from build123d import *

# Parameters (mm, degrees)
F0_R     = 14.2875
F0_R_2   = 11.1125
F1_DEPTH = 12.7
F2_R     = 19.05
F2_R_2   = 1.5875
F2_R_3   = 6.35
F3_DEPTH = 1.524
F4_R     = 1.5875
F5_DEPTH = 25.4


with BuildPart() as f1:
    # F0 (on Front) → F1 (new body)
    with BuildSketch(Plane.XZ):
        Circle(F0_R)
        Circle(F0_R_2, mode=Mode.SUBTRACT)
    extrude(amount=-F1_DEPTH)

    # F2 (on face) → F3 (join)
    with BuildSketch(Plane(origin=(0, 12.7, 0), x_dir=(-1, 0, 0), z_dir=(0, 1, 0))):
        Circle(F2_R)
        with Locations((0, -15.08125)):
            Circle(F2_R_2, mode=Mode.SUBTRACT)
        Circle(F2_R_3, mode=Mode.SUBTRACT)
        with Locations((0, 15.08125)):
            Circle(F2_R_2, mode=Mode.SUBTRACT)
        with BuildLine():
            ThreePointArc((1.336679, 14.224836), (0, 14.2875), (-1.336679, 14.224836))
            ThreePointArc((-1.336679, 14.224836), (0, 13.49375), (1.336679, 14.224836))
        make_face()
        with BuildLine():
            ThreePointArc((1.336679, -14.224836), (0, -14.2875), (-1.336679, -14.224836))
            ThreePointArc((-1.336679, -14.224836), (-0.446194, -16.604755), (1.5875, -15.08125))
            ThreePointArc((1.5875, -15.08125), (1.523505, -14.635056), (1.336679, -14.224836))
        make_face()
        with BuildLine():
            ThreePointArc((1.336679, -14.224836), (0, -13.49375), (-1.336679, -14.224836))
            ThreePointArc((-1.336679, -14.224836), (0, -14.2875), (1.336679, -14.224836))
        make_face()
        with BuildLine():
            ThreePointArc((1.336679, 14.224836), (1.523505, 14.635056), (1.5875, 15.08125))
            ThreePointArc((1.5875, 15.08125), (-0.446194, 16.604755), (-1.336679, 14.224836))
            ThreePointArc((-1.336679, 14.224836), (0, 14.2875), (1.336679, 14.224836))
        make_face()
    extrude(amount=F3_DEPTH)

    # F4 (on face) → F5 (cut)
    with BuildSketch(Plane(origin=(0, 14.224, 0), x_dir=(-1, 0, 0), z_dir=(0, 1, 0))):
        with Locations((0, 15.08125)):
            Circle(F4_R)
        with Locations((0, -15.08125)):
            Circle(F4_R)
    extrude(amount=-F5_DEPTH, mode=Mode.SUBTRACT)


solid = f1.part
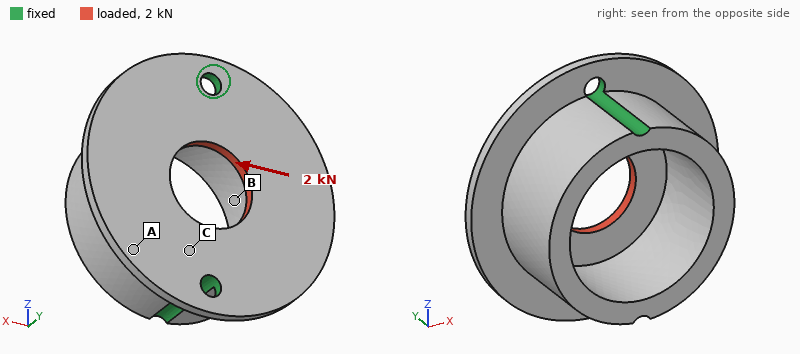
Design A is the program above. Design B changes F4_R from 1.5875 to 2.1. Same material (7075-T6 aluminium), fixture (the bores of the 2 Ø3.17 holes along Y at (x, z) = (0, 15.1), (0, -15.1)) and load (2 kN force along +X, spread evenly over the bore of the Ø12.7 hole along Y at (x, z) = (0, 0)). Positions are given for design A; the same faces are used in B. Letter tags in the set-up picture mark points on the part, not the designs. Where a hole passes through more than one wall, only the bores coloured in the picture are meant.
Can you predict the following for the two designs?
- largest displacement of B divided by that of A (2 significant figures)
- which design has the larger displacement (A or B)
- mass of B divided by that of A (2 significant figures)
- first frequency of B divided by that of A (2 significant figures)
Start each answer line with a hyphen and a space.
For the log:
- 0.91
- A
- 0.99
- 1.1
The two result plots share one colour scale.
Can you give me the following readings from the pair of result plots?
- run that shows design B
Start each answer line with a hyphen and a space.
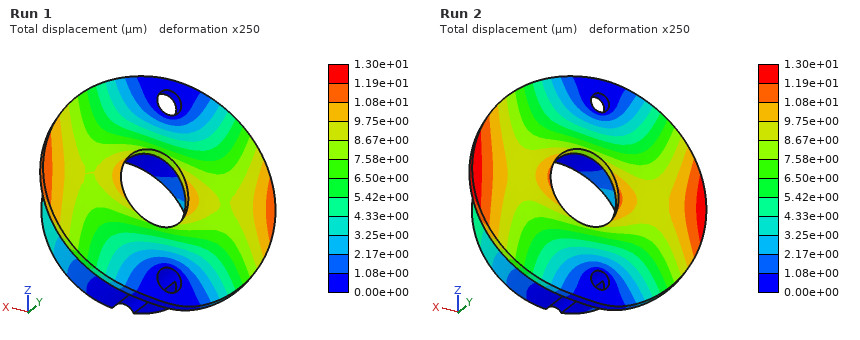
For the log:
- Run 1
